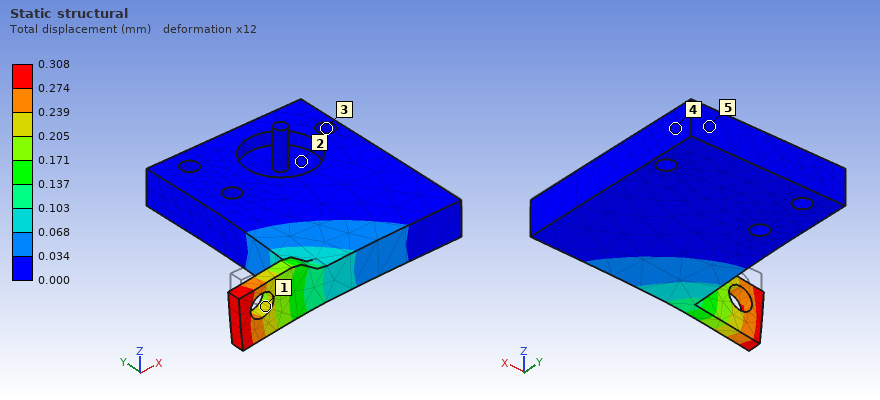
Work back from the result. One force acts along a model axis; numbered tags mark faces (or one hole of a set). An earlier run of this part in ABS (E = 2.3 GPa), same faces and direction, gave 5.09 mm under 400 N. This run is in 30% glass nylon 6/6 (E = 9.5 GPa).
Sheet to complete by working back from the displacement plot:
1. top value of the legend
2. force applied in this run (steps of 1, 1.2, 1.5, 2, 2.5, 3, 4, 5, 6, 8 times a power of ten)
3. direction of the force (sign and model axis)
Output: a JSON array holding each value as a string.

["0.308 mm", "100 N", "-Z"]
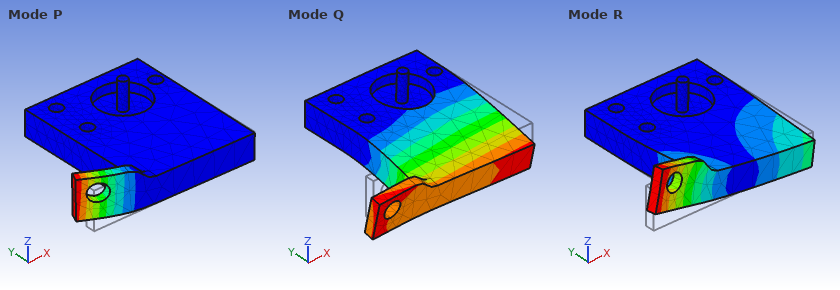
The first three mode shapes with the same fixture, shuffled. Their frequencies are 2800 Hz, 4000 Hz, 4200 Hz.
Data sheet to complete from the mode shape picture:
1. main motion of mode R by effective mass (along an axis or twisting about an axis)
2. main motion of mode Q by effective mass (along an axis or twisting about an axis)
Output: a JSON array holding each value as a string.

["twisting about Y", "along Z"]
